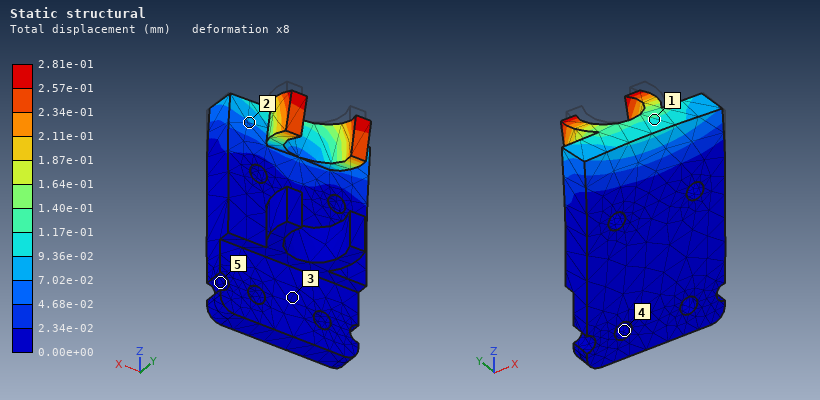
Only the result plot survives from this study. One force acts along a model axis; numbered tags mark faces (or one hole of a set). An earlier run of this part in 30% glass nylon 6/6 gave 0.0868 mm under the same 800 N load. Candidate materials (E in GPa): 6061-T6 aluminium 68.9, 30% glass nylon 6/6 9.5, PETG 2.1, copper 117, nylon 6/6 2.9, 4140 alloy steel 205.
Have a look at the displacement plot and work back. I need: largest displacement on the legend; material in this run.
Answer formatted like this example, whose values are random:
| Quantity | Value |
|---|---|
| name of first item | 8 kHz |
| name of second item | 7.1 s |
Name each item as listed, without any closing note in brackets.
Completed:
| Quantity | Value |
|---|---|
| largest displacement on the legend | 2.81e-01 mm |
| material in this run | nylon 6/6 |
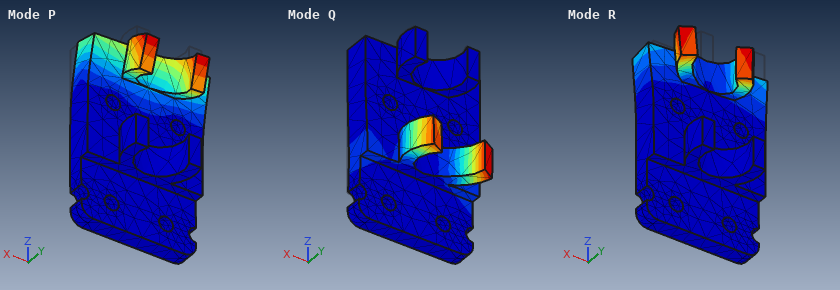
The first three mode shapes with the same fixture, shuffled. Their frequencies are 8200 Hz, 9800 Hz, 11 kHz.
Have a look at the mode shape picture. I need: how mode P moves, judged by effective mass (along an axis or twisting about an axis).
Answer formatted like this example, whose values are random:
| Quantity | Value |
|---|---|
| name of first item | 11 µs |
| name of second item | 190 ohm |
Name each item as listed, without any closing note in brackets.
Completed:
| Quantity | Value |
|---|---|
| how mode P moves, judged by effective mass | along Y |
